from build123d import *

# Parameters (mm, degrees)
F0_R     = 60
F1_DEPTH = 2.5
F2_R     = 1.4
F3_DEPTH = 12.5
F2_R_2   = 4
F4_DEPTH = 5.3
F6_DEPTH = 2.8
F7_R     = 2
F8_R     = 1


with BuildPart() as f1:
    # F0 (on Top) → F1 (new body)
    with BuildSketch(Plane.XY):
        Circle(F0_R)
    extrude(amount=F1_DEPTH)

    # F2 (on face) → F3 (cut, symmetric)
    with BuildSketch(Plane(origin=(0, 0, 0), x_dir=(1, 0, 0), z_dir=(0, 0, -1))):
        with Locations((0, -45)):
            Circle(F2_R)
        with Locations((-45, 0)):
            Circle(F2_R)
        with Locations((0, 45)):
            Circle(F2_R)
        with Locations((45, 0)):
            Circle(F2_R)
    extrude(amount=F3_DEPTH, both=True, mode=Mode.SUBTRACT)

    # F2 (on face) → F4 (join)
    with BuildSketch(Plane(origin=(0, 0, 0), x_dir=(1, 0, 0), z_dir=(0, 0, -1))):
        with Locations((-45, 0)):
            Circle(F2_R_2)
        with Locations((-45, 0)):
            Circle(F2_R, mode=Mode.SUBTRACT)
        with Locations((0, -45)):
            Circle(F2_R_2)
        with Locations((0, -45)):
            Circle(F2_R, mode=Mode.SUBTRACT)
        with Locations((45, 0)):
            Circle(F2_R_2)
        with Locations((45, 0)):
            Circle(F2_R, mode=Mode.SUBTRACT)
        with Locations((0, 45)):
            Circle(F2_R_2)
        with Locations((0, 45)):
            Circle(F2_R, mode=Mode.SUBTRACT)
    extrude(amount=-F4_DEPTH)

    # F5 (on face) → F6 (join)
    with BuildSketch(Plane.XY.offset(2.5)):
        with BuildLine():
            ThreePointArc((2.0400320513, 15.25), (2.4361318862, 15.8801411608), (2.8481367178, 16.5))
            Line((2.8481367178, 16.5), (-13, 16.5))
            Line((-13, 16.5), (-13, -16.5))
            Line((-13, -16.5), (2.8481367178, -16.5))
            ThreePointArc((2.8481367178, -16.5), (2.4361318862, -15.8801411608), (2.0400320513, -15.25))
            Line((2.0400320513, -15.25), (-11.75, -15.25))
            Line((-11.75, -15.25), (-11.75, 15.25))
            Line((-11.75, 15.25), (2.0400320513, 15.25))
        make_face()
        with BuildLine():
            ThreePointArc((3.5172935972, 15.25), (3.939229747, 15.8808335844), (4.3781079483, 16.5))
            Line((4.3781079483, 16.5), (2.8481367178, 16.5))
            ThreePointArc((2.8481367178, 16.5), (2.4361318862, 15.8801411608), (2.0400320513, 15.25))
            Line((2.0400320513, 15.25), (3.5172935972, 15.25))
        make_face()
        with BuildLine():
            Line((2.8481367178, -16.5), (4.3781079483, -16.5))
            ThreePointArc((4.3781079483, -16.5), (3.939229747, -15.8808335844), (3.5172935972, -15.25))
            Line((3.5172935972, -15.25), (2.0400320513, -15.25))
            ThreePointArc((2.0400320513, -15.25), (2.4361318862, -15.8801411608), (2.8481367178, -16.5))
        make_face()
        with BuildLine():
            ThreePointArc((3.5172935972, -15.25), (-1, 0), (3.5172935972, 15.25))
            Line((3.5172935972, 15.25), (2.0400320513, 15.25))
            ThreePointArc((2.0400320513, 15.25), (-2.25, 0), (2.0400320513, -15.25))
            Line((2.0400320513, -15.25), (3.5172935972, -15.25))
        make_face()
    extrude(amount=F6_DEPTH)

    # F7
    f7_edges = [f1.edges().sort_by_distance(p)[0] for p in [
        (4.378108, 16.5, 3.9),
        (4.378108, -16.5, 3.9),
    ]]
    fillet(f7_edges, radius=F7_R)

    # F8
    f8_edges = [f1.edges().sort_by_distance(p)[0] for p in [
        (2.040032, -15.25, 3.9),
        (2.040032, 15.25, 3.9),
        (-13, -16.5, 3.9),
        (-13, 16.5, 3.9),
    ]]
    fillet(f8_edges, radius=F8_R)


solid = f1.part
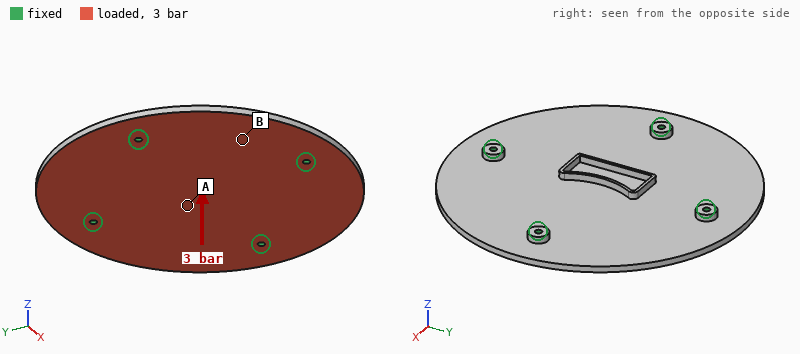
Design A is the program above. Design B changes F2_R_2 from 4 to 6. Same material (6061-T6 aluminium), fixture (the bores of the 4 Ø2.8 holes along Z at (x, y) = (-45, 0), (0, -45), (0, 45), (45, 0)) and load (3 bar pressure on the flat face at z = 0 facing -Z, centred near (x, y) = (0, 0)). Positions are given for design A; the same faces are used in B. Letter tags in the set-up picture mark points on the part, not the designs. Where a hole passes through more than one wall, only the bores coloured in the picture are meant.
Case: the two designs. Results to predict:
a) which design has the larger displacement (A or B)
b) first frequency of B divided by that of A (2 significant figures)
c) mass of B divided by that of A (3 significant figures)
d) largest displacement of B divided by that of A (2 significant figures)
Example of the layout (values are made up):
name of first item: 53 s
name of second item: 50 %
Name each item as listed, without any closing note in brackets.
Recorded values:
which design has the larger displacement: A
first frequency of B divided by that of A: 1.1
mass of B divided by that of A: 1.02
largest displacement of B divided by that of A: 0.87
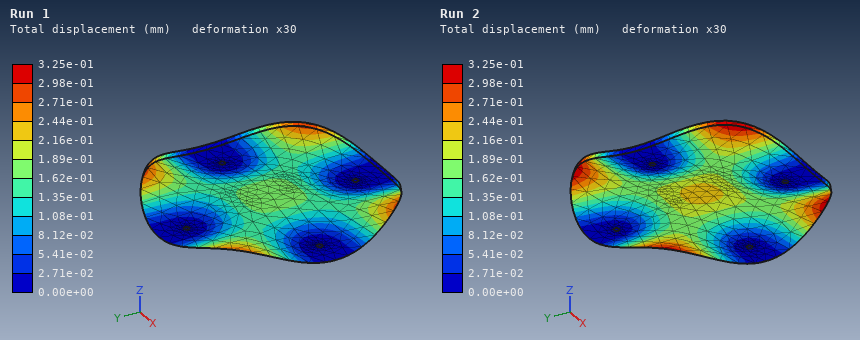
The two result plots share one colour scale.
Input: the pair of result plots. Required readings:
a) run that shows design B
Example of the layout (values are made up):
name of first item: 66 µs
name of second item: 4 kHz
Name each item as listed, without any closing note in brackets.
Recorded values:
run that shows design B: Run 1
